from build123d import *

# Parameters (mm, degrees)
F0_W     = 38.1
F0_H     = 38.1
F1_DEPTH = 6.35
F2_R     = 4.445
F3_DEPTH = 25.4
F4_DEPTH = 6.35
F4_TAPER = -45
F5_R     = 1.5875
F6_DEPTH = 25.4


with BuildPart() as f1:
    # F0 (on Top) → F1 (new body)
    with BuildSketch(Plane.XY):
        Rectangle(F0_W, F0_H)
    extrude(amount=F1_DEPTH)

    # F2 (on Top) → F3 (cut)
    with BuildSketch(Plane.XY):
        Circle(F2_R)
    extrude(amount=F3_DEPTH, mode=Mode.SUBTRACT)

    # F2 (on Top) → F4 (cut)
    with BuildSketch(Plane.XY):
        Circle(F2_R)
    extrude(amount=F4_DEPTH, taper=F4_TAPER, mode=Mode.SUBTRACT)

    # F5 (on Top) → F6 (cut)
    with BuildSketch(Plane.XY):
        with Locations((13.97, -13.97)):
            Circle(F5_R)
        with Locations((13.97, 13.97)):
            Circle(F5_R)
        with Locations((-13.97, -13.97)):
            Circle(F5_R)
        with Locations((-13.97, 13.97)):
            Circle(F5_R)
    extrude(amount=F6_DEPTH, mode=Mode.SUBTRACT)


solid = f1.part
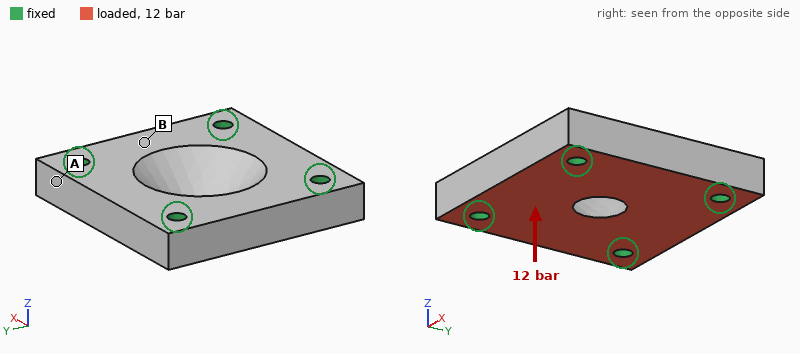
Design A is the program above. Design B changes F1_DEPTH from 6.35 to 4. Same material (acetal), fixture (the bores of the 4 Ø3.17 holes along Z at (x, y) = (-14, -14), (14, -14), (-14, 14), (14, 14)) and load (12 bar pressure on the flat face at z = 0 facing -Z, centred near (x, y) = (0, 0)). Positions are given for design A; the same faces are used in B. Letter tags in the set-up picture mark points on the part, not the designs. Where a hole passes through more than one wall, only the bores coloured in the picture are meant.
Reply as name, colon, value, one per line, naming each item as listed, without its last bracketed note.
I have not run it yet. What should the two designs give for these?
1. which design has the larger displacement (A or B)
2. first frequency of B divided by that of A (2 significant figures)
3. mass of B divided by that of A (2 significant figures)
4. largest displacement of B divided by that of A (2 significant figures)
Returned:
which design has the larger displacement: B
first frequency of B divided by that of A: 0.71
mass of B divided by that of A: 0.66
largest displacement of B divided by that of A: 2.7
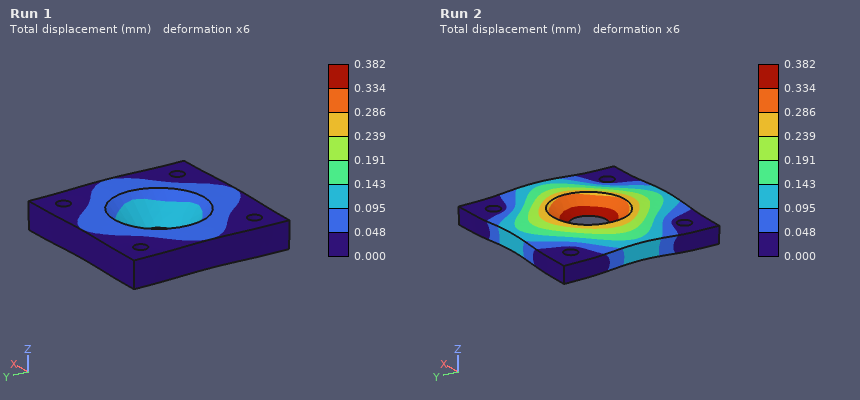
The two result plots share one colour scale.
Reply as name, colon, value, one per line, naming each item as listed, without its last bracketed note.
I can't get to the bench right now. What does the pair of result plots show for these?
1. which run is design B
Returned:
which run is design B: Run 2
